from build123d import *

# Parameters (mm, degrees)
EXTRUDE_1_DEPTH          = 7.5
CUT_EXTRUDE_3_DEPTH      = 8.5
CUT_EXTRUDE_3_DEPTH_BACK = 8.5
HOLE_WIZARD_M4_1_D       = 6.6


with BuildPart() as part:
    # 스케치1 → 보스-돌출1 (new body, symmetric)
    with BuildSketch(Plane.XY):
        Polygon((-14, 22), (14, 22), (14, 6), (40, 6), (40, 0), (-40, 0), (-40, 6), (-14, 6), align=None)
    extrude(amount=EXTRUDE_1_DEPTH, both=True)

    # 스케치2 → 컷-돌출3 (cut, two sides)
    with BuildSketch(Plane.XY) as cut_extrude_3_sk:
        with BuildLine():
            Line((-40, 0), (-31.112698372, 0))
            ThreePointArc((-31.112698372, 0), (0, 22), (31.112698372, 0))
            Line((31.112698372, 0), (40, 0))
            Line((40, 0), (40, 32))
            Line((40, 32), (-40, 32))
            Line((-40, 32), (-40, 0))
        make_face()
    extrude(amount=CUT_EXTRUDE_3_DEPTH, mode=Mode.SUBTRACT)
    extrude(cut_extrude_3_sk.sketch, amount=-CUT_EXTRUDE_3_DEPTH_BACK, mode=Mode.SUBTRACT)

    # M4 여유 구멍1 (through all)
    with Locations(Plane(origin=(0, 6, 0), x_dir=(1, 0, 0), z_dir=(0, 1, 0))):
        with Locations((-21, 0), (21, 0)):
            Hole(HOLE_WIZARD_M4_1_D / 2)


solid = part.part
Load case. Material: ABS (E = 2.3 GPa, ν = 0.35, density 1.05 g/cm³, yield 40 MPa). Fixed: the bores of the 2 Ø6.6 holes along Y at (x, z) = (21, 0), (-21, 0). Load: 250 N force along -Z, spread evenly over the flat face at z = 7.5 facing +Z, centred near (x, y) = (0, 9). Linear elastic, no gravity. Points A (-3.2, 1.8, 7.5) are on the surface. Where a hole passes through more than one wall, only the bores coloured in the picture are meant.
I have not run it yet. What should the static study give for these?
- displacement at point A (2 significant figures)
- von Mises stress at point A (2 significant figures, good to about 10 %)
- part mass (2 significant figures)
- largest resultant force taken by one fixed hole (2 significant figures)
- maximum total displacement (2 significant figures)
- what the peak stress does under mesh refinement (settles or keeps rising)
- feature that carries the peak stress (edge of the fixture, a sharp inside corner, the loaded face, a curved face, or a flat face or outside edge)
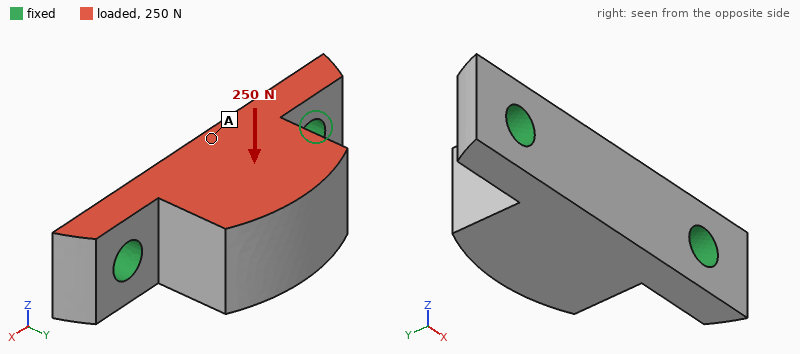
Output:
0.044 mm
1.5 MPa
12 g
130 N
0.14 mm
keeps rising
edge of the fixture
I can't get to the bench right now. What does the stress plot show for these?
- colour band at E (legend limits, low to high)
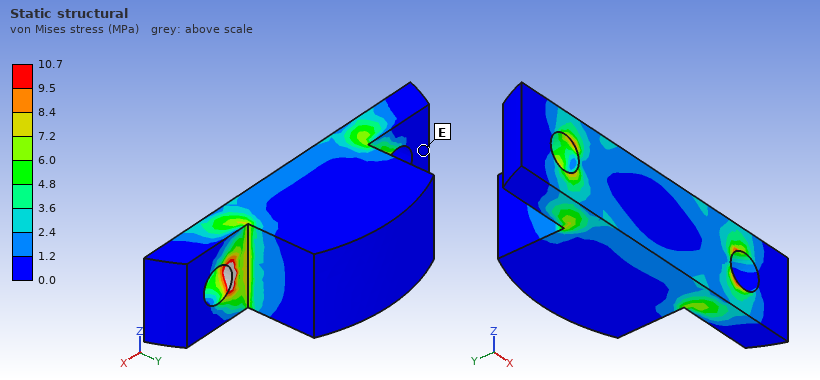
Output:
0.0 to 1.2 MPa
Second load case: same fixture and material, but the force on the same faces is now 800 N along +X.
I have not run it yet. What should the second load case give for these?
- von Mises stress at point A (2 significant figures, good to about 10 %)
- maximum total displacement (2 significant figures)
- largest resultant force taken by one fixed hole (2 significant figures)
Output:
2.3 MPa
80 µm
440 N
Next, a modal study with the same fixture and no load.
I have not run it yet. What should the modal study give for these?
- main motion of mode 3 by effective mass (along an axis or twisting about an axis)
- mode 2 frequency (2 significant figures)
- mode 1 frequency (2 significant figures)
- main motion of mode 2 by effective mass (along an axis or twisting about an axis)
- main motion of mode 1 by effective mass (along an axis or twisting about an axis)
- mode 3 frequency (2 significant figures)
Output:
along X
5100 Hz
2300 Hz
along Y
along Z
6300 Hz
